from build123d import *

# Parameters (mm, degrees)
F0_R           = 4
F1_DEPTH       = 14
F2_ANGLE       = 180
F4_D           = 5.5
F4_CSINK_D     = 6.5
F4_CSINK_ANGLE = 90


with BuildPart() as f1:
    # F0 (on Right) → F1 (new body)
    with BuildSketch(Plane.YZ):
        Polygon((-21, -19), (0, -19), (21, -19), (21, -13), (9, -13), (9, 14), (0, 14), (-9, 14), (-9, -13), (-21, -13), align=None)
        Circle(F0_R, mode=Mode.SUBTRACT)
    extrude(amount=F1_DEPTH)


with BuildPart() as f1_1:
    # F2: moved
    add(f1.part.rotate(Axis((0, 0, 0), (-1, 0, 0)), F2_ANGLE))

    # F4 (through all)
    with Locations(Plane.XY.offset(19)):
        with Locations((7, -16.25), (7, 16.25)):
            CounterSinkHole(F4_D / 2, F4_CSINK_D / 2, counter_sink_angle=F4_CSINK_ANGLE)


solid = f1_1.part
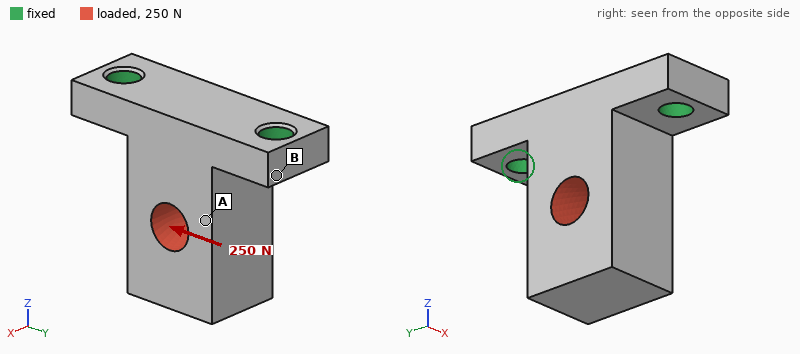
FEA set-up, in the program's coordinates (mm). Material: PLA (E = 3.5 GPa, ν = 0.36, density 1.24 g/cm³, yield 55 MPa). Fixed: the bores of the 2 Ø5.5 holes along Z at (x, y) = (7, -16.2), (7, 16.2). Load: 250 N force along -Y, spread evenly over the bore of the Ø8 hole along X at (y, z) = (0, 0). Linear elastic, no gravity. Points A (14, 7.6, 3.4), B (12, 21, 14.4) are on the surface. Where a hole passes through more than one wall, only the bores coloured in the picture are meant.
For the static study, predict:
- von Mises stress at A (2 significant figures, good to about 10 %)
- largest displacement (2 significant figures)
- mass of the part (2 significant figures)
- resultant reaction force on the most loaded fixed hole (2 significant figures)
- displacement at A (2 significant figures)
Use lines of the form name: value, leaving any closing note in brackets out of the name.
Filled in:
von Mises stress at A: 2.1 MPa
largest displacement: 0.11 mm
mass of the part: 12 g
resultant reaction force on the most loaded fixed hole: 210 N
displacement at A: 0.046 mm
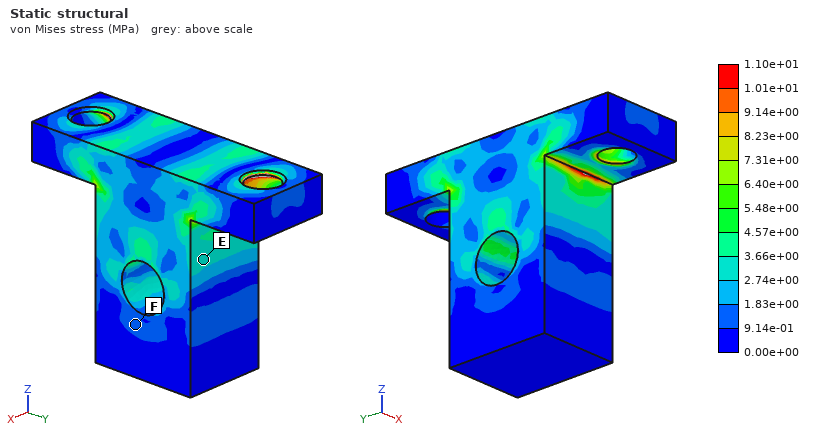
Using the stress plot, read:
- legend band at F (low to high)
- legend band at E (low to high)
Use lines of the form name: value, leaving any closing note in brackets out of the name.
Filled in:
legend band at F: 9.14e-01 to 1.83e+00 MPa
legend band at E: 2.74e+00 to 3.66e+00 MPa
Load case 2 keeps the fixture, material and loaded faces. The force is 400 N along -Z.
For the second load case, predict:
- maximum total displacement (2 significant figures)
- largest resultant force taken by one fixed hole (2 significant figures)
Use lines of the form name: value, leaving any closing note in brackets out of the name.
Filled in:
maximum total displacement: 41 µm
largest resultant force taken by one fixed hole: 210 N
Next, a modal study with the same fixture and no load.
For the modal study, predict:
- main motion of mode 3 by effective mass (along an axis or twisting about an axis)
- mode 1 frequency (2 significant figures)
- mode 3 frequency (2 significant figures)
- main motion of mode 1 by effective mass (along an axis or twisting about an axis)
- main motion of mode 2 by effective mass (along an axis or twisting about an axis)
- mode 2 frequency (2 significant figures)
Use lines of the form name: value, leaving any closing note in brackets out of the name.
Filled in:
main motion of mode 3 by effective mass: along Z
mode 1 frequency: 1500 Hz
mode 3 frequency: 5500 Hz
main motion of mode 1 by effective mass: along X
main motion of mode 2 by effective mass: along Y
mode 2 frequency: 3100 Hz
